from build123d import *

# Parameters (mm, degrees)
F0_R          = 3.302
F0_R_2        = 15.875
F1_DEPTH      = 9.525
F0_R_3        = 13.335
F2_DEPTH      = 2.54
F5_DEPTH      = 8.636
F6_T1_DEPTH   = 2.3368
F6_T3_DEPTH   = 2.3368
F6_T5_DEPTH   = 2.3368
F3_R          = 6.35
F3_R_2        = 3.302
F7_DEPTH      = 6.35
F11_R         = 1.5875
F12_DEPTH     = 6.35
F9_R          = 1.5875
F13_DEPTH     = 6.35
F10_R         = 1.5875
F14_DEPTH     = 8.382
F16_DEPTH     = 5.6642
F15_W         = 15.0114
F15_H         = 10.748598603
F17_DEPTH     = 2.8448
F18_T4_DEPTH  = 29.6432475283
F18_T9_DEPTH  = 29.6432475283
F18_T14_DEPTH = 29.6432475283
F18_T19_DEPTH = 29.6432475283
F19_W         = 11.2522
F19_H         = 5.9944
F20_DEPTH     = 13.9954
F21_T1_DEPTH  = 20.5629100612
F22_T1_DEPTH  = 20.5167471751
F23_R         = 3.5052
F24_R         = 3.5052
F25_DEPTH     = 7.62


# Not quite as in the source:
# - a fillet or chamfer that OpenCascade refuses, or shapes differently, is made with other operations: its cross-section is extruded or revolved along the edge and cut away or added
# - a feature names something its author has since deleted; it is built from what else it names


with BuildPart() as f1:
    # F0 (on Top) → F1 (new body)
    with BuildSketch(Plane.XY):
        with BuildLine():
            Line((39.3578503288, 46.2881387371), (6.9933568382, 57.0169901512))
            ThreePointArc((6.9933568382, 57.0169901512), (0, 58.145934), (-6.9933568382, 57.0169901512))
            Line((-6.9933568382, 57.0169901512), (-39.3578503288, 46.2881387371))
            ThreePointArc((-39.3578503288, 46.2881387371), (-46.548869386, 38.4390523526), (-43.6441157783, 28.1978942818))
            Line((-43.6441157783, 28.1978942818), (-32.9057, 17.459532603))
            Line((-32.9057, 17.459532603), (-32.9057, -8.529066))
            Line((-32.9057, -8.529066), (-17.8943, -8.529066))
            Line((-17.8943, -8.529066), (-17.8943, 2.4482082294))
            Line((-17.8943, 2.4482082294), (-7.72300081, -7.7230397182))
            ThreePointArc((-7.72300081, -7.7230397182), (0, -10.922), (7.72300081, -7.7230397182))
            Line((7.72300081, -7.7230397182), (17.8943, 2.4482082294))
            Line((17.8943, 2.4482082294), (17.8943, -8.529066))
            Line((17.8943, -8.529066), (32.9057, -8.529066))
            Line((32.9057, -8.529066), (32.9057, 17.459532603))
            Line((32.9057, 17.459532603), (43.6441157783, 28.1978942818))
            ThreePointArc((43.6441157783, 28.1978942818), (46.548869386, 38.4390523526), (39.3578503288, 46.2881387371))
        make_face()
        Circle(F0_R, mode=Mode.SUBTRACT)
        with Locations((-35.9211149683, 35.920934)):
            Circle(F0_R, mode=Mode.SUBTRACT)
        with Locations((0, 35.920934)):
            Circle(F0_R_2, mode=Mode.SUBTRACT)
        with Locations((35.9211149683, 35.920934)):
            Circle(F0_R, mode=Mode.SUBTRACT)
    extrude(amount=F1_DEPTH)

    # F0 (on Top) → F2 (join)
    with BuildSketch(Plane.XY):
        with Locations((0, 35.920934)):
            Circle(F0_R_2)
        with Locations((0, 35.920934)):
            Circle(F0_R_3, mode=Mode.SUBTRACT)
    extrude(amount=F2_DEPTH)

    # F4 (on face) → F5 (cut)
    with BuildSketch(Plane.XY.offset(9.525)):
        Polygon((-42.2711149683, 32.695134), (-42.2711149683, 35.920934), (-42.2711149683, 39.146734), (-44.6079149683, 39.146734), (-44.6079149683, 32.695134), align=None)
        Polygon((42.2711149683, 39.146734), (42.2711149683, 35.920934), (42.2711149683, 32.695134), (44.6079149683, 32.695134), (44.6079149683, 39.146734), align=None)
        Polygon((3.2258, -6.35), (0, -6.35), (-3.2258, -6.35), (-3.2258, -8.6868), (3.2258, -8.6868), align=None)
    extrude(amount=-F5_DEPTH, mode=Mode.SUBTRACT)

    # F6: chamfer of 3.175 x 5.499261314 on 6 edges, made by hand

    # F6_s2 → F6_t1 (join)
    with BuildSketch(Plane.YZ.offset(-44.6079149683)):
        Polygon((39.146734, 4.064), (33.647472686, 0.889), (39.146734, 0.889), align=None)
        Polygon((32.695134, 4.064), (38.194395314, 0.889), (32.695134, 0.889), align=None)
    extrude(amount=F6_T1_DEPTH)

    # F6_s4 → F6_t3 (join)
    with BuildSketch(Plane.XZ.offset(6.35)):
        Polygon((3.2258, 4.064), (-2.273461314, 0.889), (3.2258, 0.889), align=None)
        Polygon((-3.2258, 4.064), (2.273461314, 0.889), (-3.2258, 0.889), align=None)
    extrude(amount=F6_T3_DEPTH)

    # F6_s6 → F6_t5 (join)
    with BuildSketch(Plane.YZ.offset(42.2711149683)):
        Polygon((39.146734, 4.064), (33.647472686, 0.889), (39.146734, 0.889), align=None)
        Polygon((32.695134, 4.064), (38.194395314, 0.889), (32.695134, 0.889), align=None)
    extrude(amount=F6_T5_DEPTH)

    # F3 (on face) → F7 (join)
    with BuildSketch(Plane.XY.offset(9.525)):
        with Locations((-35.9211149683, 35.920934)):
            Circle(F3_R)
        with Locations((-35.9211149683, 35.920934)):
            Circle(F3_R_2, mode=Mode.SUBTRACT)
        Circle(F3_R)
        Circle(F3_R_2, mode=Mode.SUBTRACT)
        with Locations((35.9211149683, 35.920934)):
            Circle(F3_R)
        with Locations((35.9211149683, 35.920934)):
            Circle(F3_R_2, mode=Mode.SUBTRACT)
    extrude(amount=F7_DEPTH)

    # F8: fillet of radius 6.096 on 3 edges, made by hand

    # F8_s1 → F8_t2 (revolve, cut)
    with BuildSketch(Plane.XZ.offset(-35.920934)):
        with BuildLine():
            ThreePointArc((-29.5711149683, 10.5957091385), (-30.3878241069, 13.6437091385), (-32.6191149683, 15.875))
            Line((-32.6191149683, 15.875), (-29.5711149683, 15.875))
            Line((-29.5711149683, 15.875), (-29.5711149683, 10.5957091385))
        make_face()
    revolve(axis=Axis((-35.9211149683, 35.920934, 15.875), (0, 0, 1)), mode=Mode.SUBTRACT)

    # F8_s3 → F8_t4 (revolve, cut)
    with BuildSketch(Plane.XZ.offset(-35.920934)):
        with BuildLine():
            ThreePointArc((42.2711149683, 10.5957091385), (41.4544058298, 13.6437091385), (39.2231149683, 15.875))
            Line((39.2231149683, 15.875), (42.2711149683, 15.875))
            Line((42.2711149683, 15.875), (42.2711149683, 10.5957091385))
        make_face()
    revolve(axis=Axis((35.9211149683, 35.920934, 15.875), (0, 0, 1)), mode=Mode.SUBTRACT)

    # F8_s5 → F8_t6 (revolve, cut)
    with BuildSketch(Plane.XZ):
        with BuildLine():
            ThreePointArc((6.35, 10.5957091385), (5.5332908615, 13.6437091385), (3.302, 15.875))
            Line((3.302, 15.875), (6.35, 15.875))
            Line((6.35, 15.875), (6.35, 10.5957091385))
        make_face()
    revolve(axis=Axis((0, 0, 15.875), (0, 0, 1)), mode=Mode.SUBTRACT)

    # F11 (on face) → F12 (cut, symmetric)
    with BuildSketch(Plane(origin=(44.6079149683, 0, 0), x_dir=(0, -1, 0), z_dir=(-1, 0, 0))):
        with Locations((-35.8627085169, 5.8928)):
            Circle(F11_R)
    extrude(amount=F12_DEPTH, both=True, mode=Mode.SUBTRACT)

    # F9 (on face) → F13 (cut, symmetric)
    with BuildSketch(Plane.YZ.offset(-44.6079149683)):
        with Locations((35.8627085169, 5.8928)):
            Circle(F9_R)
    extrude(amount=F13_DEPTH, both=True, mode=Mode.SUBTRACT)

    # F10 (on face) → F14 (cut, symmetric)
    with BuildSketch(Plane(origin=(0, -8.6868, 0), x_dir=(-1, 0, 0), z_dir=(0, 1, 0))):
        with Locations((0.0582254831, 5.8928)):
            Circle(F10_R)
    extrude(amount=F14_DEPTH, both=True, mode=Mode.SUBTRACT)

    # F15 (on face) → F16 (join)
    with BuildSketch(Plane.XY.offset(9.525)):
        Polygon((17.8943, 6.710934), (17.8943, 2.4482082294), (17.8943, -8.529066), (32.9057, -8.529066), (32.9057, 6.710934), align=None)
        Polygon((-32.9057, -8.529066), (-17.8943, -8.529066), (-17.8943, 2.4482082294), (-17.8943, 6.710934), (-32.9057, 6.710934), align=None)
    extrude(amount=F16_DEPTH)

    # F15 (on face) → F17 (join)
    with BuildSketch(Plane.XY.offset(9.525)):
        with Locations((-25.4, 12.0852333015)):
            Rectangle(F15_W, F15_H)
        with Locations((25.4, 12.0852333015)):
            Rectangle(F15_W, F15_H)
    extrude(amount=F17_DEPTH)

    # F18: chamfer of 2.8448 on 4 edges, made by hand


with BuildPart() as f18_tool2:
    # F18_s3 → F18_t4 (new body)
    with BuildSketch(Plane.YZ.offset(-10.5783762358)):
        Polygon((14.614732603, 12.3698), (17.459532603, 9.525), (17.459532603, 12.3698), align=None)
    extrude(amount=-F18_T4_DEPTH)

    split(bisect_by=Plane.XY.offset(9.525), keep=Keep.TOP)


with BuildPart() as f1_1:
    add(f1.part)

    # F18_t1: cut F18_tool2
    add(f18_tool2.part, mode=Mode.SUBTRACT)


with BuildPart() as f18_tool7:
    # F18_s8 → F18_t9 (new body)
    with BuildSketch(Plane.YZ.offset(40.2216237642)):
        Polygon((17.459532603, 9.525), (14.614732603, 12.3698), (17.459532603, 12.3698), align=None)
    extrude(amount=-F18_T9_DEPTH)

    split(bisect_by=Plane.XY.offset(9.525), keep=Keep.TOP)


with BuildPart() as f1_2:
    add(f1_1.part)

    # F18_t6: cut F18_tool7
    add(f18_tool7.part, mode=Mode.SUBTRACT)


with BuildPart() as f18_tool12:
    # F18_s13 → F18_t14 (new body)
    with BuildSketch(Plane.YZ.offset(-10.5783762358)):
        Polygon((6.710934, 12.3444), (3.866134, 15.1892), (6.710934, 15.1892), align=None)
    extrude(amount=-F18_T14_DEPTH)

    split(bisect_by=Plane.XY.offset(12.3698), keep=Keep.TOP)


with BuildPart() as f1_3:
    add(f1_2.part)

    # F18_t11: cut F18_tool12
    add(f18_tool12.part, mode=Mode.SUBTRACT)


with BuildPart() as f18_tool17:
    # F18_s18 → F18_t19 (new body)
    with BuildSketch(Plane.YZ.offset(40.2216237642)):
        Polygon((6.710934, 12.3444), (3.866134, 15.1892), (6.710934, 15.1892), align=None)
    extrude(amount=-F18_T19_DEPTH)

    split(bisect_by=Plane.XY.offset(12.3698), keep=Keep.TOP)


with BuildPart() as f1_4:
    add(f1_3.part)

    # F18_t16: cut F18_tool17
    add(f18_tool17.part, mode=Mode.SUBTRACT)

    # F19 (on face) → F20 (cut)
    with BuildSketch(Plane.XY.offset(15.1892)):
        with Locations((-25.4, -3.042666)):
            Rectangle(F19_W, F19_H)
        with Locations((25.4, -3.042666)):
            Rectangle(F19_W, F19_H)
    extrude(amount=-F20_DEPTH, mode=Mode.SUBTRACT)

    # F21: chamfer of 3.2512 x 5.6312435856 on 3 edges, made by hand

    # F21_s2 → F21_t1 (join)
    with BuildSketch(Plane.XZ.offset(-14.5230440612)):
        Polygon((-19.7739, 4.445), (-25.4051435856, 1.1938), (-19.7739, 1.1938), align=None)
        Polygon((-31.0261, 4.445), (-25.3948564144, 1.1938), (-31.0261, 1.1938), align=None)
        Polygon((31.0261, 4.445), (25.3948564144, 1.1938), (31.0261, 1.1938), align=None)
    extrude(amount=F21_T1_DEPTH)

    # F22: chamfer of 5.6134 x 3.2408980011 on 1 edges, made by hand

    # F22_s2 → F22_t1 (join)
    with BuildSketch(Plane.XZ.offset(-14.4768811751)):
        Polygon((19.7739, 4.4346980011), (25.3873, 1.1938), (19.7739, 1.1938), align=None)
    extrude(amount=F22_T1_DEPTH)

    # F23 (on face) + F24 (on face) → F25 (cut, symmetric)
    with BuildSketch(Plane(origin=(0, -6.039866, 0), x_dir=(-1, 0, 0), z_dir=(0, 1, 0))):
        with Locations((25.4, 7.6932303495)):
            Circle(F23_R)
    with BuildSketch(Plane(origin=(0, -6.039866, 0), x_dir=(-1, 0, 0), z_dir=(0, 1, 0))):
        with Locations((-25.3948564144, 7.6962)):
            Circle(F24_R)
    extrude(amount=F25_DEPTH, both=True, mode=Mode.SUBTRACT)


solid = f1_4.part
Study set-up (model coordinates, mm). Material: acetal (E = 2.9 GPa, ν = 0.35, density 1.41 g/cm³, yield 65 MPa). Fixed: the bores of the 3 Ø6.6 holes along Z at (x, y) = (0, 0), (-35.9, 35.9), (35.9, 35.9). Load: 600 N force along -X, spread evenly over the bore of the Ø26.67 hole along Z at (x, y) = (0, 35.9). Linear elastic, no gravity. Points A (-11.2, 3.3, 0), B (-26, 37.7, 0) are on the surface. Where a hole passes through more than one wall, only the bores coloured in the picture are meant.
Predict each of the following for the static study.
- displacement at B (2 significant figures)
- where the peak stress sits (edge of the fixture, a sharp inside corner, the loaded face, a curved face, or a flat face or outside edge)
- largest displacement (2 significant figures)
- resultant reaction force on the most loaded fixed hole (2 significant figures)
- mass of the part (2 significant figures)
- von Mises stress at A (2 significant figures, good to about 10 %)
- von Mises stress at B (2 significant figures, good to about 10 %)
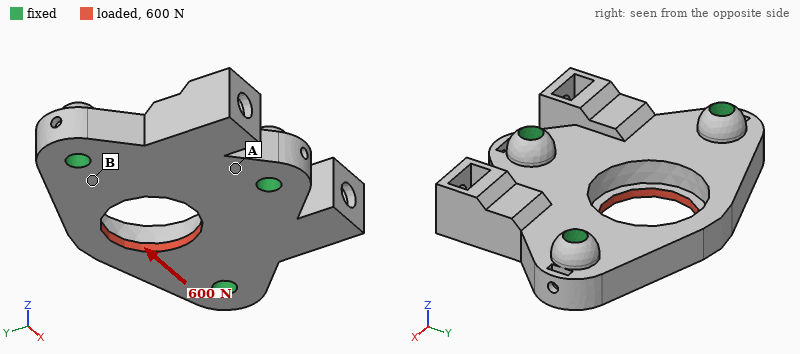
5.6 µm
a sharp inside corner
29 µm
250 N
53 g
0.62 MPa
2.2 MPa
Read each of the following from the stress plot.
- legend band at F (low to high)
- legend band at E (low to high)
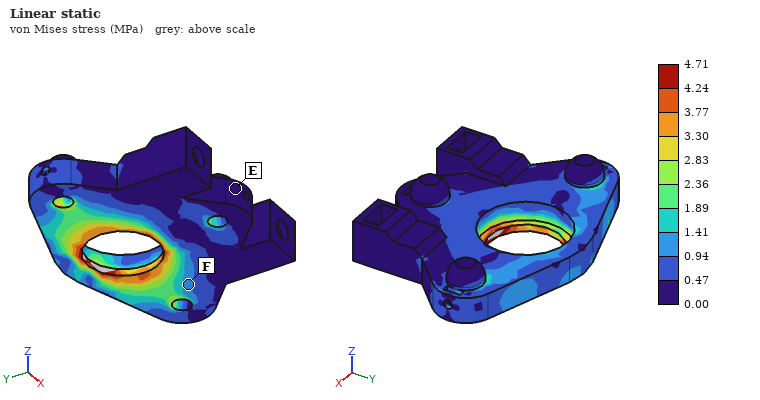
0.94 to 1.41 MPa
0.00 to 0.47 MPa
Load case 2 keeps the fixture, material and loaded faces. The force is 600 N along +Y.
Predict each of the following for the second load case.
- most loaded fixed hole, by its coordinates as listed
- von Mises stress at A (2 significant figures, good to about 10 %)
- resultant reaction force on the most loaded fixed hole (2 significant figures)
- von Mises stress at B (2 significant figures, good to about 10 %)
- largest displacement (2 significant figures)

(0, 0)
1.0 MPa
260 N
1.9 MPa
86 µm
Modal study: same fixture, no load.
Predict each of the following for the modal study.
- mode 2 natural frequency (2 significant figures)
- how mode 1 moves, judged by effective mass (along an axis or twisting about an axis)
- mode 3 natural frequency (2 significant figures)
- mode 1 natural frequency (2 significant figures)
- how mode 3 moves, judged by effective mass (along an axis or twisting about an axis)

2600 Hz
twisting about X
2800 Hz
2400 Hz
along Z
